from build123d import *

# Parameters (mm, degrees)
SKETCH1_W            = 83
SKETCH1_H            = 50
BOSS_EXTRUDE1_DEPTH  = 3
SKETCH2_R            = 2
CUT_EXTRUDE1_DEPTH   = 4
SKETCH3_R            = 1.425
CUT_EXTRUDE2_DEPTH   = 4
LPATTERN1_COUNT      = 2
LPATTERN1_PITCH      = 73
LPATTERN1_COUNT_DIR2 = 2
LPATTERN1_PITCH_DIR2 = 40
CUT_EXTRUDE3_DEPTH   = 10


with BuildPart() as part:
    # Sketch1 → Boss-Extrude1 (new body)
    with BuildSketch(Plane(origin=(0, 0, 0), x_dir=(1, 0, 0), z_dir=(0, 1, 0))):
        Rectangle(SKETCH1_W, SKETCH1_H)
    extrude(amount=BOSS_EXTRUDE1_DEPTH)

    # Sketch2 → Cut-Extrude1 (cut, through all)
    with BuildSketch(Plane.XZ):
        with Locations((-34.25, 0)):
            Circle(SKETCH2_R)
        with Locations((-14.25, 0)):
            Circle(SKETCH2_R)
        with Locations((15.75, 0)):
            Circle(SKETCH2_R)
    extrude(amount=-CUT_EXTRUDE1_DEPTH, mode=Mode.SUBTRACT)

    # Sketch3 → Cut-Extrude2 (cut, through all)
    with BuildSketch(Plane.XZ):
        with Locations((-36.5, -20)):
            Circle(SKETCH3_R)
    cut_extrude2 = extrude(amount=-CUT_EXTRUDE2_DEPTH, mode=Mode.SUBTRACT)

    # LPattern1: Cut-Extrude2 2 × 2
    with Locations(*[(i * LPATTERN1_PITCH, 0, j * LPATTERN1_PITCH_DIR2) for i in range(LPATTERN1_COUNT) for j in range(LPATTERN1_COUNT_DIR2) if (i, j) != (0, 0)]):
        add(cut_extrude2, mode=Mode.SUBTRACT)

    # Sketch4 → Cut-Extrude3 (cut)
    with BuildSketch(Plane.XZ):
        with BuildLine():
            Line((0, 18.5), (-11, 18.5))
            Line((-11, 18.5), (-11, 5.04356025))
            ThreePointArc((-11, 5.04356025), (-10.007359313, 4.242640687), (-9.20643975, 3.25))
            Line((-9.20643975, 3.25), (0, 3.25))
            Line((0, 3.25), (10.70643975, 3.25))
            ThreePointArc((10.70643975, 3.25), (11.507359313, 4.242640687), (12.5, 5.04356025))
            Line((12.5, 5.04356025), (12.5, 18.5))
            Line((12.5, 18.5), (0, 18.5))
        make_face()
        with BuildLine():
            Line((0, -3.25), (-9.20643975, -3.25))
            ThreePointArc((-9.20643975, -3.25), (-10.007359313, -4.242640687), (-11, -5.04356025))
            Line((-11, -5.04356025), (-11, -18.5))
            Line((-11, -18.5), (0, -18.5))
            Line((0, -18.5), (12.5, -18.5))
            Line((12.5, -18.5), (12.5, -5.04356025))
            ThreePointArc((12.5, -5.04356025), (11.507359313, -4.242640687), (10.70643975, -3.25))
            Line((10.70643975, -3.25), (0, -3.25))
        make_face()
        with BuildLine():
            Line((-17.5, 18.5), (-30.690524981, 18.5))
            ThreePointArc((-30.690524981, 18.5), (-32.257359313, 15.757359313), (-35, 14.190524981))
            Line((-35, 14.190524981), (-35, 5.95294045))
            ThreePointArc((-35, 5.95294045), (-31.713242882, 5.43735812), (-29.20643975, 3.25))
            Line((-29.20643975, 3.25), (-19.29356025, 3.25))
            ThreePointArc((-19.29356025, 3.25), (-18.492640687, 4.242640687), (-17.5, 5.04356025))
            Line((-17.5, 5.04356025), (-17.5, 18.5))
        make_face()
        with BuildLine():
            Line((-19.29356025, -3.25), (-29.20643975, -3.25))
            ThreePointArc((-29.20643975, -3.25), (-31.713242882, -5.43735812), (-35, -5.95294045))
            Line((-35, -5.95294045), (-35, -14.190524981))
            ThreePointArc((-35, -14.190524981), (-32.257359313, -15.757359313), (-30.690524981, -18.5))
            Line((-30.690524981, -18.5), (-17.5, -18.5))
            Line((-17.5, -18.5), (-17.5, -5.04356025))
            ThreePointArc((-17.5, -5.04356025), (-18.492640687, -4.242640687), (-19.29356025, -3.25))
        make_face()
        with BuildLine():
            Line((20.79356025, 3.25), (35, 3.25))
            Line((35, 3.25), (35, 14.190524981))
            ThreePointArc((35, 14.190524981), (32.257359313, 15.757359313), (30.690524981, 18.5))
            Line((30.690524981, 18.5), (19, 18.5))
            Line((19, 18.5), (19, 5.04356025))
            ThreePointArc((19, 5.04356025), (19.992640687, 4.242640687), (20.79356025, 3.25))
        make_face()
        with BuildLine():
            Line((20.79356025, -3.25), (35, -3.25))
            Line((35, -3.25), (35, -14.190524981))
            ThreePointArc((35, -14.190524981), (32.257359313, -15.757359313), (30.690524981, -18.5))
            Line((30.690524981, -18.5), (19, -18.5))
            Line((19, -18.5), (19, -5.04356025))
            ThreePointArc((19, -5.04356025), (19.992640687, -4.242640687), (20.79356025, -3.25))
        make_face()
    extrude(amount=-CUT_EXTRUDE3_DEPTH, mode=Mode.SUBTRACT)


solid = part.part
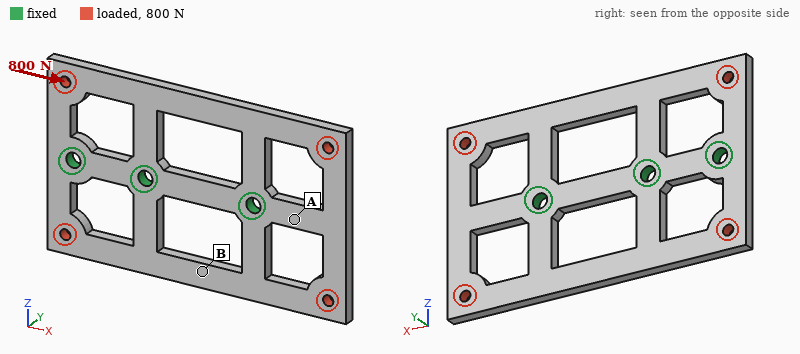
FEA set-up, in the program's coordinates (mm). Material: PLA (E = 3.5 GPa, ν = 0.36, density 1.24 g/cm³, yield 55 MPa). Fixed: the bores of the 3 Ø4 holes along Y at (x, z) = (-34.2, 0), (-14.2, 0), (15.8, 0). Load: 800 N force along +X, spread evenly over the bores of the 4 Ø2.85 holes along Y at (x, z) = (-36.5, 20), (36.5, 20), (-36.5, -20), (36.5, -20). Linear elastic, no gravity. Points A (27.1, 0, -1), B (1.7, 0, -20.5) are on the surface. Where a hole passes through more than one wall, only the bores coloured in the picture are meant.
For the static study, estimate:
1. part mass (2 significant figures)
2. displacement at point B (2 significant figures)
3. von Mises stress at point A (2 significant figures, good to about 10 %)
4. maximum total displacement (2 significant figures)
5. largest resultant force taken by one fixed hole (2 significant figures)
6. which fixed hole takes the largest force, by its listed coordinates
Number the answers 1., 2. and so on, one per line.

1. 9.1 g
2. 0.29 mm
3. 9.2 MPa
4. 0.35 mm
5. 370 N
6. (15.8, 0)
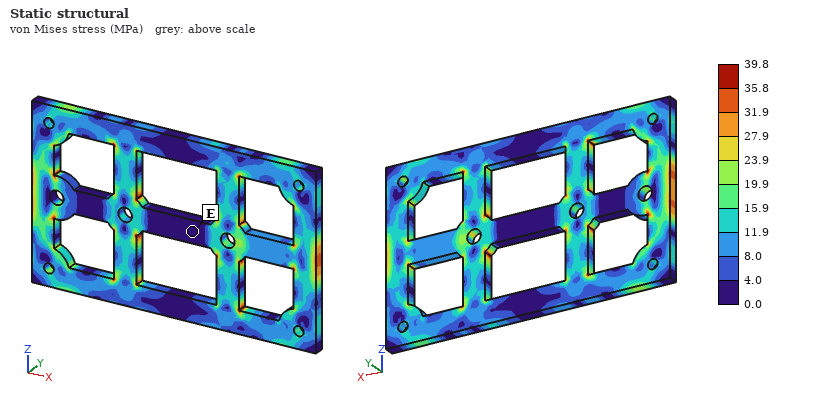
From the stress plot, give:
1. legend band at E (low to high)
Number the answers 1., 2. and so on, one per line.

1. 0.0 to 4.0 MPa
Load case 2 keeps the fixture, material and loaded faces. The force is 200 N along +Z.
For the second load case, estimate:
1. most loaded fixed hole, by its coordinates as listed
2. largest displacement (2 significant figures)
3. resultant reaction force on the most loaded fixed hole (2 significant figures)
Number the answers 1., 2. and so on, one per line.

1. (15.8, 0)
2. 0.22 mm
3. 120 N
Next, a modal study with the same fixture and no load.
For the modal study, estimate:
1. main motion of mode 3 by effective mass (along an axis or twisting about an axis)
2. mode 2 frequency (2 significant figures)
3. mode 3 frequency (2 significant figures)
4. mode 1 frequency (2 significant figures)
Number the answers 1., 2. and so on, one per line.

1. along Y
2. 710 Hz
3. 950 Hz
4. 680 Hz
